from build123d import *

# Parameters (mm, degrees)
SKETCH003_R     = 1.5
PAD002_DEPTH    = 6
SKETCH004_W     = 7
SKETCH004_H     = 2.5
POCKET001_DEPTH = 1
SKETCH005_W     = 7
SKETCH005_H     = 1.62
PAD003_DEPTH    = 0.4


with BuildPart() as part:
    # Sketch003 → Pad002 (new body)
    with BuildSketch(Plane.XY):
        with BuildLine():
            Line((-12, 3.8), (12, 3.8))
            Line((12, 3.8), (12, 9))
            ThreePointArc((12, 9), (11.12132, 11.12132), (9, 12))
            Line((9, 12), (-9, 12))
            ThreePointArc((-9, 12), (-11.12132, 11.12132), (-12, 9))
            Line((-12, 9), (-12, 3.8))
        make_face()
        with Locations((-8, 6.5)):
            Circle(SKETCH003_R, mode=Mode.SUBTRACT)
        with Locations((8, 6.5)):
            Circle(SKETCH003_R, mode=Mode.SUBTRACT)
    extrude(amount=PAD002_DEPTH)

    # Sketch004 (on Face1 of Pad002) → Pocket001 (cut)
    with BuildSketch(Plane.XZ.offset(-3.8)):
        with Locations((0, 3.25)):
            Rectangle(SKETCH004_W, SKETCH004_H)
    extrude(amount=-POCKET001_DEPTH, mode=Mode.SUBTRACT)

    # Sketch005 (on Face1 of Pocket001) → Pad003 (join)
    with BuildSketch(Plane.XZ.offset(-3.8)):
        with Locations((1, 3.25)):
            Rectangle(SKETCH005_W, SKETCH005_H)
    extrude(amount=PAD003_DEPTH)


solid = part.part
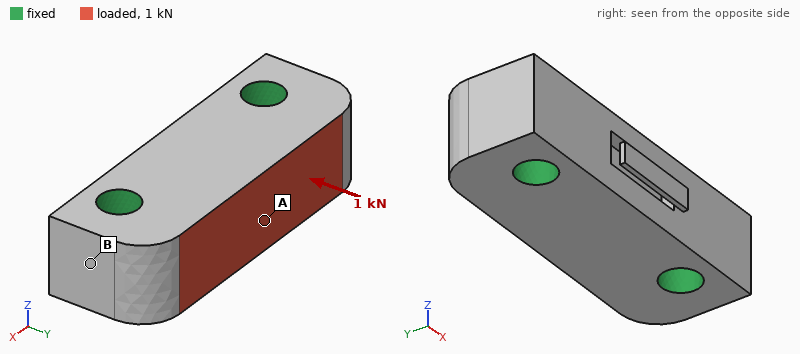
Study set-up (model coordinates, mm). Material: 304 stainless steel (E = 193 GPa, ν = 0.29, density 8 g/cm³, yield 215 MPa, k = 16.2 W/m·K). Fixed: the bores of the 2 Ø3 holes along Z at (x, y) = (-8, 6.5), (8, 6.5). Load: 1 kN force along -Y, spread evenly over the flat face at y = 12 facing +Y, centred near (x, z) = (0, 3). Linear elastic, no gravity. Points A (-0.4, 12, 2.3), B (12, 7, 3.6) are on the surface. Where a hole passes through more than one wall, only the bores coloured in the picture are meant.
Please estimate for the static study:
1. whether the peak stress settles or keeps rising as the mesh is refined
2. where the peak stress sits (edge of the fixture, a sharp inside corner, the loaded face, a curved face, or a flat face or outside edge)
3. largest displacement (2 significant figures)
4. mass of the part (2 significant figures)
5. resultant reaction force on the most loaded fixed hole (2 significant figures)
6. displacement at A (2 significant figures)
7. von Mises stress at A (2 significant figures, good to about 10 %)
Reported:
keeps rising
edge of the fixture
1.2 µm
8.5 g
530 N
0.83 µm
15 MPa
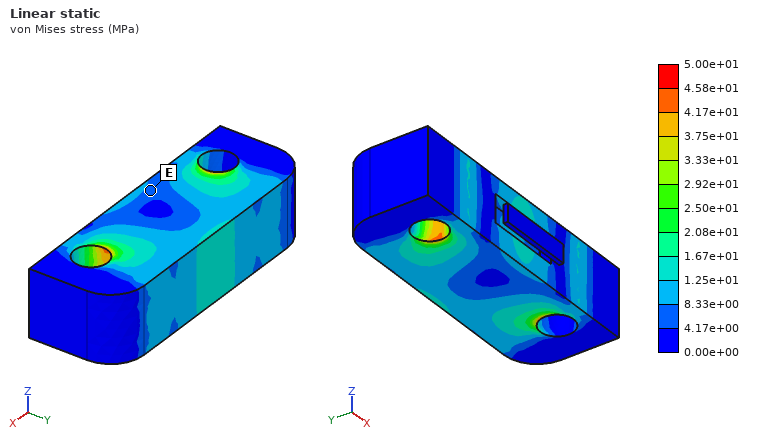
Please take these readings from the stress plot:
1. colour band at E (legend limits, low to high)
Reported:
4.17e+00 to 8.33e+00 MPa
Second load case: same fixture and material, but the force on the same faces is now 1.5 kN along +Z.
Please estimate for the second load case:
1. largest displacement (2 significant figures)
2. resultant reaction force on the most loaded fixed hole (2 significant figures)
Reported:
5.0 µm
750 N
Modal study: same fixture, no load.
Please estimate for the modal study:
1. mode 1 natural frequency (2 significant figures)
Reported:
8200 Hz
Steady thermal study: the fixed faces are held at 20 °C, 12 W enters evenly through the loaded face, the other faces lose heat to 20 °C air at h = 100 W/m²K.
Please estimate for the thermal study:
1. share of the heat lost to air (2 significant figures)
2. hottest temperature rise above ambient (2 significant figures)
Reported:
6.8 %
47 K
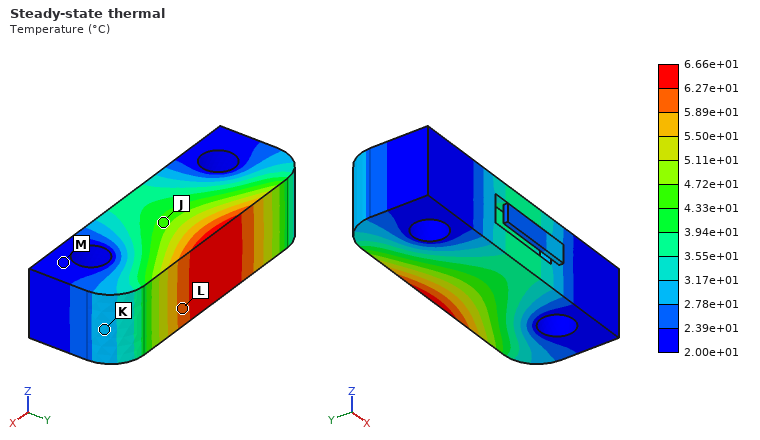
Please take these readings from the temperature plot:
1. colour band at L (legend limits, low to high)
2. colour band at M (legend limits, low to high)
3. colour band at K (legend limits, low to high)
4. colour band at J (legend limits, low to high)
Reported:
5.89e+01 to 6.27e+01 °C
2.00e+01 to 2.39e+01 °C
2.78e+01 to 3.17e+01 °C
4.33e+01 to 4.72e+01 °C
